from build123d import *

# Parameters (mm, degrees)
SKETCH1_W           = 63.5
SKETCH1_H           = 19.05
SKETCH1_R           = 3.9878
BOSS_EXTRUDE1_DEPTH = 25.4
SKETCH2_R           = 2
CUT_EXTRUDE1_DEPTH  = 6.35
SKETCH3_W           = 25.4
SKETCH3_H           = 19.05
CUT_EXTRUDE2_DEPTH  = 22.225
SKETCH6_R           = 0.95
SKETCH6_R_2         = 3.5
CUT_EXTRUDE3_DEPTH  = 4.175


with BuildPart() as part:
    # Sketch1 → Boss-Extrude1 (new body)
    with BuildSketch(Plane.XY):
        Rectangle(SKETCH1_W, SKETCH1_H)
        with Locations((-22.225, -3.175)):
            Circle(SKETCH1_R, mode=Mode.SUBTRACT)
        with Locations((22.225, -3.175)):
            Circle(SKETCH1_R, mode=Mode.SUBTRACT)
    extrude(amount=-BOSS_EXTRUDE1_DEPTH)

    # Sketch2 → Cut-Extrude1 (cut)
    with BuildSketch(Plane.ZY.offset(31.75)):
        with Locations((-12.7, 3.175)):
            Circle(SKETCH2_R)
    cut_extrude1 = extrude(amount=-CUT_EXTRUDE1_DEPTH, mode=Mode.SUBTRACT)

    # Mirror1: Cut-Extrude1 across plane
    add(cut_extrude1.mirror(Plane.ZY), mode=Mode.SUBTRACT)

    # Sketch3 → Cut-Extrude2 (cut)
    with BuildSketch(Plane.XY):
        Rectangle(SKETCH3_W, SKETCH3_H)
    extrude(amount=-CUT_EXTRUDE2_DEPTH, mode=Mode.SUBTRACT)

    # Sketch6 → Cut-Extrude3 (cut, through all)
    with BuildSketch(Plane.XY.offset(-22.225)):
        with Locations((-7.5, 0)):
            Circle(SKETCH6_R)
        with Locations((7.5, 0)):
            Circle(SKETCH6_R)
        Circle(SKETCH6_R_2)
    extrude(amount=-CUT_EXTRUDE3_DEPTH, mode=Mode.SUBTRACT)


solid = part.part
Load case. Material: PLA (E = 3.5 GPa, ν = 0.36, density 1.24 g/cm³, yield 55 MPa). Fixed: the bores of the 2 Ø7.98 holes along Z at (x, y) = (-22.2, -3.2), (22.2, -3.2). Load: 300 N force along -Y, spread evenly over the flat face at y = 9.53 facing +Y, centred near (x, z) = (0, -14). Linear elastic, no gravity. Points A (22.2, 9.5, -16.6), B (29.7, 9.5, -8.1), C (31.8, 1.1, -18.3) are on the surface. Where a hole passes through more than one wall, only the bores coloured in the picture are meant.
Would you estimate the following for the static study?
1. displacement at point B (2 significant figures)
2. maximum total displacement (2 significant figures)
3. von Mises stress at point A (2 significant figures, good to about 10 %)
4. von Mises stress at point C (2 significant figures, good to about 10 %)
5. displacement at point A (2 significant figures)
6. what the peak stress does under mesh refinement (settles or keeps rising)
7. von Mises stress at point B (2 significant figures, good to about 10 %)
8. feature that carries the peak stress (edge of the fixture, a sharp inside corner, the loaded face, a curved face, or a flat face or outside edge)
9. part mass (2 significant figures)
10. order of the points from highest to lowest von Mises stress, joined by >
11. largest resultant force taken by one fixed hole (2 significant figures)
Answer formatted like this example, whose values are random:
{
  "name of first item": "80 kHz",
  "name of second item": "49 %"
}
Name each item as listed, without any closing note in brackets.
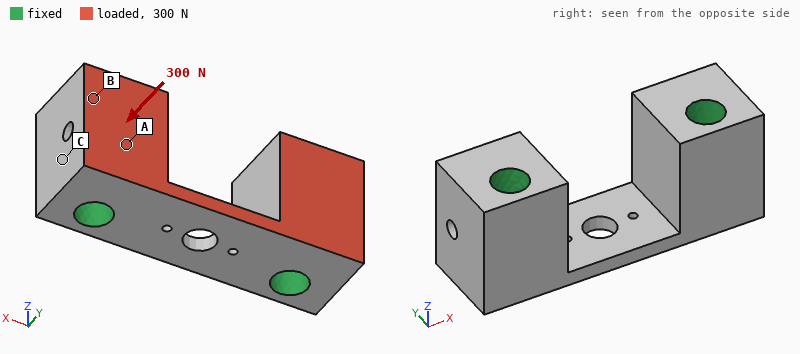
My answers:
{
  "displacement at point B": "1.2 µm",
  "maximum total displacement": "4.1 µm",
  "von Mises stress at point A": "0.45 MPa",
  "von Mises stress at point C": "0.16 MPa",
  "displacement at point A": "0.94 µm",
  "what the peak stress does under mesh refinement": "keeps rising",
  "von Mises stress at point B": "0.30 MPa",
  "feature that carries the peak stress": "edge of the fixture",
  "part mass": "21 g",
  "order of the points from highest to lowest von Mises stress, joined by >": "A > B > C",
  "largest resultant force taken by one fixed hole": "150 N"
}
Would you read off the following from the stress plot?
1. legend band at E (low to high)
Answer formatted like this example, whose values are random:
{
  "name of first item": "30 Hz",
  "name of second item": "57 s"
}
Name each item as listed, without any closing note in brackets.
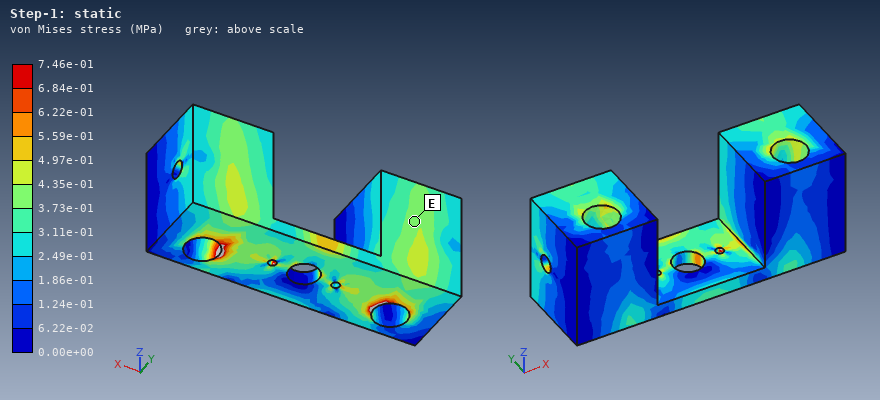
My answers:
{
  "legend band at E": "3.73e-01 to 4.35e-01 MPa"
}
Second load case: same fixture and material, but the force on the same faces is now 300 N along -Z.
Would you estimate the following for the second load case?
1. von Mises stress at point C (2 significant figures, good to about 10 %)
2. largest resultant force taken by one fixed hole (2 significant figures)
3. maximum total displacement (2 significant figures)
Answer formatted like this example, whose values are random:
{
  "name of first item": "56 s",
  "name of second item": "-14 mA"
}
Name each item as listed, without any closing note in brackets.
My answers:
{
  "von Mises stress at point C": "0.29 MPa",
  "largest resultant force taken by one fixed hole": "150 N",
  "maximum total displacement": "39 µm"
}
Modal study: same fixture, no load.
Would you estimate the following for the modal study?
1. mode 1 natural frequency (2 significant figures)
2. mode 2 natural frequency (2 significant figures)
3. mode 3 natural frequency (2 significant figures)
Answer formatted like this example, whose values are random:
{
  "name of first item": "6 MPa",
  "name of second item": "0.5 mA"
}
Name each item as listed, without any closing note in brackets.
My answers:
{
  "mode 1 natural frequency": "6400 Hz",
  "mode 2 natural frequency": "8100 Hz",
  "mode 3 natural frequency": "12 kHz"
}
